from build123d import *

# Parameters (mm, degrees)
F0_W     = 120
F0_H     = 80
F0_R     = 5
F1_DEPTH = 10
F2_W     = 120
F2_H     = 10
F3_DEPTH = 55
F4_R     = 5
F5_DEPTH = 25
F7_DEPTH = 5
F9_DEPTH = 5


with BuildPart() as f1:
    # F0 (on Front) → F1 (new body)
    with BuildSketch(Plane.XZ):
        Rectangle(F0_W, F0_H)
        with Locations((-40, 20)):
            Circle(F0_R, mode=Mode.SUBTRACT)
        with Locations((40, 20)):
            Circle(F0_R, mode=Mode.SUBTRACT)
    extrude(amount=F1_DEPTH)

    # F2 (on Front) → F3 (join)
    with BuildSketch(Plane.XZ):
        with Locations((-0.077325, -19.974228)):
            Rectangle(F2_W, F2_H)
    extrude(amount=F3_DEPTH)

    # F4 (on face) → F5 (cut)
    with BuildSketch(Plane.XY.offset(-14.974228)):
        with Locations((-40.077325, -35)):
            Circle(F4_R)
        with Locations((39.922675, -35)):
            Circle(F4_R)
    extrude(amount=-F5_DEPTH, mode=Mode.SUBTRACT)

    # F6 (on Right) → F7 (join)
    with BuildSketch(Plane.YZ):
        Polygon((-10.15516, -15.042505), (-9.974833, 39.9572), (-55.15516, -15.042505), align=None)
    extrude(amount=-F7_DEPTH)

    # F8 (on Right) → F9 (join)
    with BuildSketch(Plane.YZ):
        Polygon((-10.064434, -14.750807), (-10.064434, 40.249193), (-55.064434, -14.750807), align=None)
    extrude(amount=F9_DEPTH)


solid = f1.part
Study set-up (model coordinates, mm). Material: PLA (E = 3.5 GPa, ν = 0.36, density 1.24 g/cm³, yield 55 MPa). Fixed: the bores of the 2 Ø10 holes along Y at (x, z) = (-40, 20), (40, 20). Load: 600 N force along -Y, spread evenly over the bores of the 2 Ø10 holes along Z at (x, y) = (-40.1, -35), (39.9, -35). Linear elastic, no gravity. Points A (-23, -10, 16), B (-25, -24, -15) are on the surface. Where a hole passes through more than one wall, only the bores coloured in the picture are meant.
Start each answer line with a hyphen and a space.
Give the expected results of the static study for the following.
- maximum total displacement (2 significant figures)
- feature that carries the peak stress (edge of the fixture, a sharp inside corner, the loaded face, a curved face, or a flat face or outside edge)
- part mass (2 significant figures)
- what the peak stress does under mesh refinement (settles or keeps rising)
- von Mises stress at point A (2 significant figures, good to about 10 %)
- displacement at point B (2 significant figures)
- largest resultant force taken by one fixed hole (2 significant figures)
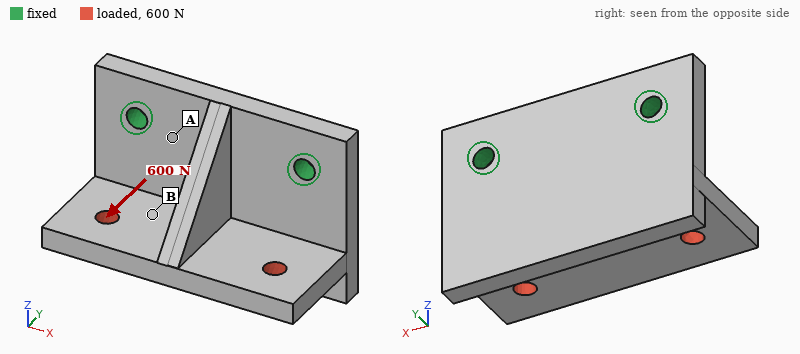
- 0.71 mm
- edge of the fixture
- 200 g
- keeps rising
- 5.0 MPa
- 0.39 mm
- 300 N
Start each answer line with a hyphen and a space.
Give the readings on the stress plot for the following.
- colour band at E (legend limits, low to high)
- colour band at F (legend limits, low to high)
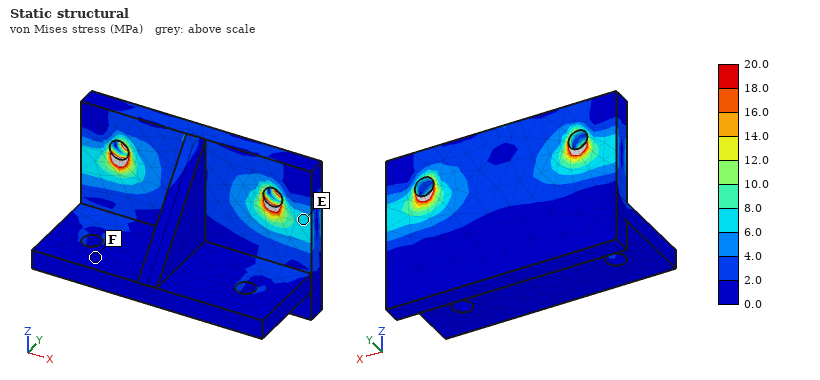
- 6.0 to 8.0 MPa
- 0.0 to 2.0 MPa
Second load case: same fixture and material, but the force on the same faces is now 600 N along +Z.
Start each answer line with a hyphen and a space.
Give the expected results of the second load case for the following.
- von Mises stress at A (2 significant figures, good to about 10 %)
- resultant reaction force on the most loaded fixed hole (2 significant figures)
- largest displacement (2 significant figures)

- 4.8 MPa
- 300 N
- 0.93 mm
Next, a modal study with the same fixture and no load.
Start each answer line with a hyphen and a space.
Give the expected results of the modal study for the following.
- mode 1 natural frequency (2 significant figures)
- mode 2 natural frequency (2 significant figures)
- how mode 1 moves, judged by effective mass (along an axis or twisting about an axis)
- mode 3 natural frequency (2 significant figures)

- 450 Hz
- 740 Hz
- along Y
- 1400 Hz
